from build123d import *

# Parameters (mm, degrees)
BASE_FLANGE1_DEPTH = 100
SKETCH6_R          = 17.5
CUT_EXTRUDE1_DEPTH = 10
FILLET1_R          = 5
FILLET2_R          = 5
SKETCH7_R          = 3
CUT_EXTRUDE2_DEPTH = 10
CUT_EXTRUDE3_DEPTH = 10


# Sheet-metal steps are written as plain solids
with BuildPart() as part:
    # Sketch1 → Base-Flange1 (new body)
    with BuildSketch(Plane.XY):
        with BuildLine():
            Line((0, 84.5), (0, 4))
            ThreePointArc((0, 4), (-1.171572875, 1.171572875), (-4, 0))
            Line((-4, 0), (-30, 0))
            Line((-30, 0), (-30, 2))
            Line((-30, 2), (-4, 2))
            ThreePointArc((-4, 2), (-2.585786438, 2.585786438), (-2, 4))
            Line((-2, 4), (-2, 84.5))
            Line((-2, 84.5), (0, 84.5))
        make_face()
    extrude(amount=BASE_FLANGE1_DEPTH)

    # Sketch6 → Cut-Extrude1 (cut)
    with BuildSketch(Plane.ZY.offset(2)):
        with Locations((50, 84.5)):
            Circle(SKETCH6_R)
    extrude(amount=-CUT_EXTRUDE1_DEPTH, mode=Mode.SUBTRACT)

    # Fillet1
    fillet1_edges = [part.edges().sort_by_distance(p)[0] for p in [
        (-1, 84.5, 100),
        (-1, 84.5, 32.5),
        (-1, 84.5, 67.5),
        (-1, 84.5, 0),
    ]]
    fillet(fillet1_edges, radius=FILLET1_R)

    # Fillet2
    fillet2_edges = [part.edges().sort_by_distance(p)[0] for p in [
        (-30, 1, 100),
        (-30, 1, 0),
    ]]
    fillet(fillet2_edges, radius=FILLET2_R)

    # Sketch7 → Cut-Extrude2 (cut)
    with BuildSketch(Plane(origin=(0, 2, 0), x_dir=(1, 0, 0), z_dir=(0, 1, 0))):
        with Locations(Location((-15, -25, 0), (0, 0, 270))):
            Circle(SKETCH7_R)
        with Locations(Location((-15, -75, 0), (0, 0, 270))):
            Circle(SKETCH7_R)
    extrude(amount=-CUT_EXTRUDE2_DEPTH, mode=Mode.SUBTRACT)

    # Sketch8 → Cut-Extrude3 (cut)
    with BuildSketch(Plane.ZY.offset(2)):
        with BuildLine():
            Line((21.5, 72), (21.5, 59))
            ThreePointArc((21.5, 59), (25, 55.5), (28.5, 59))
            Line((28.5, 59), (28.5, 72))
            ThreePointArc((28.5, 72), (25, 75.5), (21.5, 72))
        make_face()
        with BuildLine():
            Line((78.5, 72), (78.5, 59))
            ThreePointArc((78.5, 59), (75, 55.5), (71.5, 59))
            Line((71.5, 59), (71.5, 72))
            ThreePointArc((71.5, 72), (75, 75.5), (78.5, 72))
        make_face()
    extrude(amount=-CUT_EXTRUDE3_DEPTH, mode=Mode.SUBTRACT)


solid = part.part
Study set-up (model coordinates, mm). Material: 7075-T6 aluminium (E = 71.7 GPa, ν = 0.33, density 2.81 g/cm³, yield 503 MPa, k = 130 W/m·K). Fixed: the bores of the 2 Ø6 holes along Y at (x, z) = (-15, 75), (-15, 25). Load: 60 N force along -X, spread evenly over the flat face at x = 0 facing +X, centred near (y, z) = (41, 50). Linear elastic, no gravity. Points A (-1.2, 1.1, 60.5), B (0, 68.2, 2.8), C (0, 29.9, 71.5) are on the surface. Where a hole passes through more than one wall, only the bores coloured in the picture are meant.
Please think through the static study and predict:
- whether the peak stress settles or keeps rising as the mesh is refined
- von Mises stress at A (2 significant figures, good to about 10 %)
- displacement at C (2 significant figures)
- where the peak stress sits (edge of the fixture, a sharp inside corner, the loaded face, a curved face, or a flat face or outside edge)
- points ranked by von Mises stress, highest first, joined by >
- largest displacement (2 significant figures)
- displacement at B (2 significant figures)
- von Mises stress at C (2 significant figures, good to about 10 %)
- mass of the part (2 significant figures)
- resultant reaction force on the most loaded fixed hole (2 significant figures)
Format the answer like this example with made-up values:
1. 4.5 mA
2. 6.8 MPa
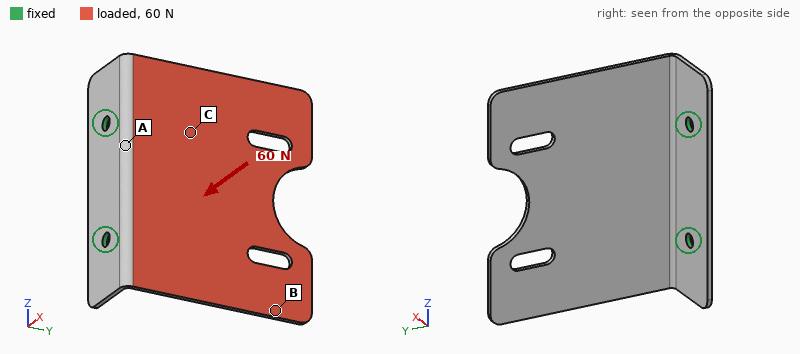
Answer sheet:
1. keeps rising
2. 28 MPa
3. 0.35 mm
4. edge of the fixture
5. A > C > B
6. 1.3 mm
7. 1.0 mm
8. 13 MPa
9. 58 g
10. 30 N
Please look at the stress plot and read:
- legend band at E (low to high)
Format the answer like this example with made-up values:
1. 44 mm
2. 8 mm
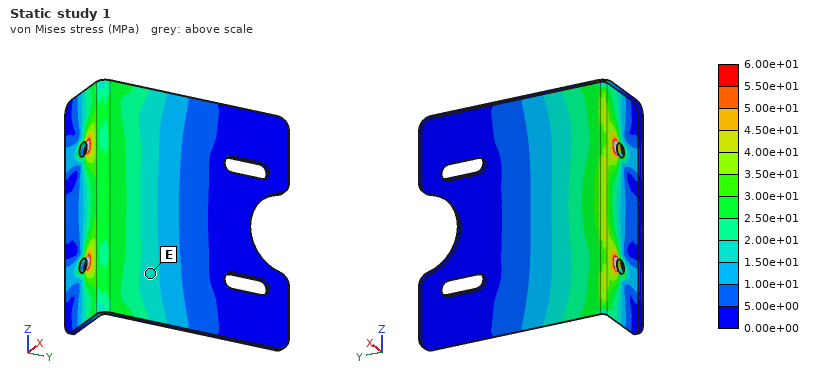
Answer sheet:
1. 1.50e+01 to 2.00e+01 MPa
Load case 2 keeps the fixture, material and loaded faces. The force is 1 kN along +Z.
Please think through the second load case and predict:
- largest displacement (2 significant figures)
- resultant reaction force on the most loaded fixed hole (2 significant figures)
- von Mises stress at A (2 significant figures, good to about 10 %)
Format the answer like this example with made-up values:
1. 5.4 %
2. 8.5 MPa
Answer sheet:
1. 1.1 mm
2. 930 N
3. 58 MPa
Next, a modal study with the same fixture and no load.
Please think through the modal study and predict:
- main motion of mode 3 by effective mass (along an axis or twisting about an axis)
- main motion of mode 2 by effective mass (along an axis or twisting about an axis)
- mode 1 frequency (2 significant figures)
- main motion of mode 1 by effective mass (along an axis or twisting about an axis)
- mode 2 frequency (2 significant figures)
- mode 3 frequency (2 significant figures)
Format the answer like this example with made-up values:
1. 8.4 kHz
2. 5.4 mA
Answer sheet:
1. along Z
2. twisting about Y
3. 210 Hz
4. along X
5. 430 Hz
6. 970 Hz
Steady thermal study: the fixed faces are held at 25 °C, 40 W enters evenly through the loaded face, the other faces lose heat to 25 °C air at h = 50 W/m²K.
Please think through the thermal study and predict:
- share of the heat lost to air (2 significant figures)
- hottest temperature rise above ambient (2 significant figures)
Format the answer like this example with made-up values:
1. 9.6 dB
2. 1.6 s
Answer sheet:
1. 48 %
2. 51 K
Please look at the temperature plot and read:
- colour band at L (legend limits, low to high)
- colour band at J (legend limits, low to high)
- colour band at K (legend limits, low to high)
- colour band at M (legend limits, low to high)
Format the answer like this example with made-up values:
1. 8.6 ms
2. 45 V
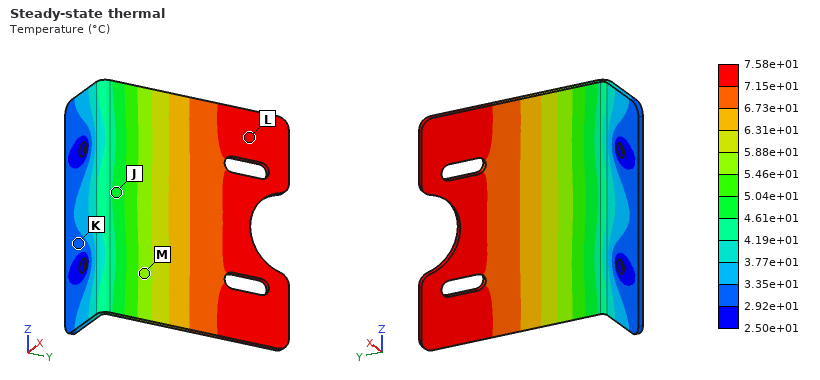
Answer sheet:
1. 7.15e+01 to 7.58e+01 °C
2. 4.61e+01 to 5.04e+01 °C
3. 2.92e+01 to 3.35e+01 °C
4. 5.46e+01 to 5.88e+01 °C
